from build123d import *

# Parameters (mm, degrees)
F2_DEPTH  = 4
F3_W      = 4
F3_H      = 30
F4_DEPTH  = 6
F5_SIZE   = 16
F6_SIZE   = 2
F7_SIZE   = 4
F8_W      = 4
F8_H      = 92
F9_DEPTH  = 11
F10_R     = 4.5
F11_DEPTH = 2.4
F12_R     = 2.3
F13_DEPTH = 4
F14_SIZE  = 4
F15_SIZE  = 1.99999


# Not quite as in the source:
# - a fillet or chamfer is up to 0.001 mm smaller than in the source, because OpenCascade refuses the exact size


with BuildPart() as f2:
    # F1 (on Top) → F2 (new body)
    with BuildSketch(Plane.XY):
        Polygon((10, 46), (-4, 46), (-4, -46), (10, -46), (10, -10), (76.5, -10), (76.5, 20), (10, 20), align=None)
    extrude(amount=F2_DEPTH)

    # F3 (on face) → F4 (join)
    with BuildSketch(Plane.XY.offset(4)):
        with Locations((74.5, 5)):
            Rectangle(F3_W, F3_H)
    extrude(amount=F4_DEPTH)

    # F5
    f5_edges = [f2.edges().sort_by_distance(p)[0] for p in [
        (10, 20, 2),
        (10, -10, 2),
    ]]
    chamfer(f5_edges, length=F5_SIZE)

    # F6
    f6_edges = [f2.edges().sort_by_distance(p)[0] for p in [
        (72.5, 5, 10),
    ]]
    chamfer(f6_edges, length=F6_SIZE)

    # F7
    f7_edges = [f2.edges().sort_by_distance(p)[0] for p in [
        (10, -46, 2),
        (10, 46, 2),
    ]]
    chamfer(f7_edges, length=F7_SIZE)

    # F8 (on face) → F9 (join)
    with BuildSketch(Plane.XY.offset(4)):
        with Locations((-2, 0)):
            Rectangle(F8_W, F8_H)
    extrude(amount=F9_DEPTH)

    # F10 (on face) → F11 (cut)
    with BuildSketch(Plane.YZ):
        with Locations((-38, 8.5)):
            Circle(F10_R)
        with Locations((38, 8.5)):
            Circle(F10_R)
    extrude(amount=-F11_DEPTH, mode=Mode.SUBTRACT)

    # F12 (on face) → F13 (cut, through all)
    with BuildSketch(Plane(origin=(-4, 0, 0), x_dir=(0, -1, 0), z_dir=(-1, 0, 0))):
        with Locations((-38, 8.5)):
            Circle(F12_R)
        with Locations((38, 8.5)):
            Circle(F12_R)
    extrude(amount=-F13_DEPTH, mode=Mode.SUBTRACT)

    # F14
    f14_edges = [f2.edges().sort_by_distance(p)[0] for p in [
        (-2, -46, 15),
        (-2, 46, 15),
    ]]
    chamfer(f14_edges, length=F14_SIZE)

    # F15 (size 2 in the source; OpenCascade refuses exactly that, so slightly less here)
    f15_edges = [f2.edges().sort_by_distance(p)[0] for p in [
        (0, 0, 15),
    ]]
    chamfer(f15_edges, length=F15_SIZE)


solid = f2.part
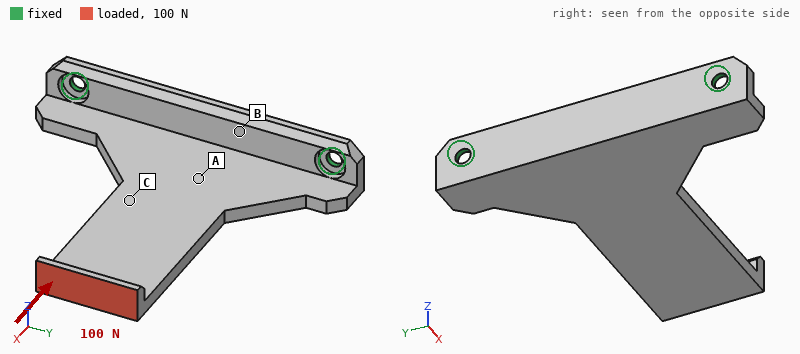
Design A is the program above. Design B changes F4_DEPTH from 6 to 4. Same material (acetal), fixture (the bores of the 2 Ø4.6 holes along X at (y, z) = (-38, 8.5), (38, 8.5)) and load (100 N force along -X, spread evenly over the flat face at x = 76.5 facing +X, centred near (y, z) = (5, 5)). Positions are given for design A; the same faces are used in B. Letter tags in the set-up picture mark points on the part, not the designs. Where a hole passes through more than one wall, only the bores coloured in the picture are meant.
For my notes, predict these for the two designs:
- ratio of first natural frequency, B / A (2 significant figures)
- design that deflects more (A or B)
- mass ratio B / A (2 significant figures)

1.0
A
0.99
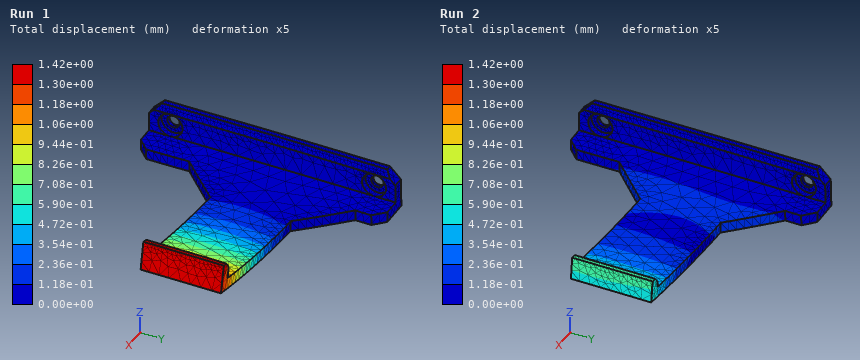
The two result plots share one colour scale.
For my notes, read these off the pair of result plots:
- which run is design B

Run 2
